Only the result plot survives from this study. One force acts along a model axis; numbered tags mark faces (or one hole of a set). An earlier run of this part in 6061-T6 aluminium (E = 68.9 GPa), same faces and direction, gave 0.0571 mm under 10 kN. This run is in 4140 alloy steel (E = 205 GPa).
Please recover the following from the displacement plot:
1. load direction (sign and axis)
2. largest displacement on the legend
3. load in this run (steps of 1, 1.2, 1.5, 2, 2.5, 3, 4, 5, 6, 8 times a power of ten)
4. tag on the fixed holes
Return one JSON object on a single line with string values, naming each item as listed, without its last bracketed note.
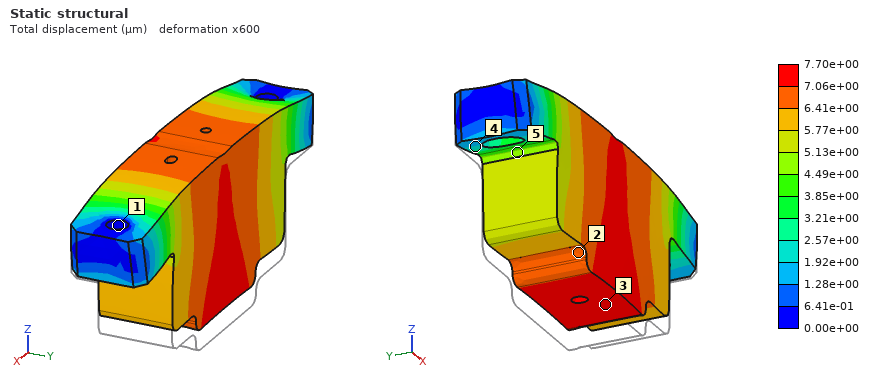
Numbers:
{"load direction": "+Z", "largest displacement on the legend": "7.70e+00 µm", "load in this run": "4 kN", "tag on the fixed holes": "1"}
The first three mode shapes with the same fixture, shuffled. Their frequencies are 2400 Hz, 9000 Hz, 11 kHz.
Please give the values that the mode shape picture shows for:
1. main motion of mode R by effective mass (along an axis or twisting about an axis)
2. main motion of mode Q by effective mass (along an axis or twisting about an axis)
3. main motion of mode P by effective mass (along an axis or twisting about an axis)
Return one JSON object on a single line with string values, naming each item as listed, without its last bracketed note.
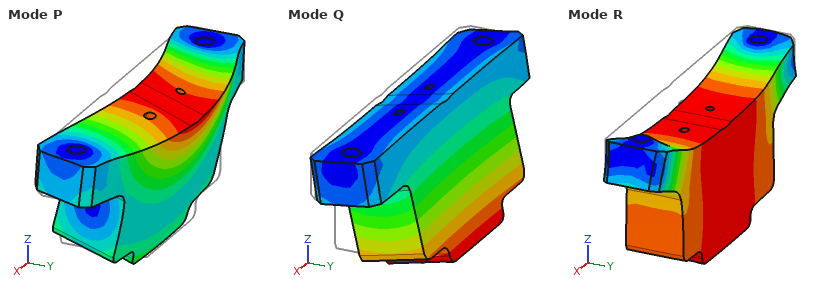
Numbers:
{"main motion of mode R by effective mass": "along Z", "main motion of mode Q by effective mass": "along Y", "main motion of mode P by effective mass": "along Y"}
